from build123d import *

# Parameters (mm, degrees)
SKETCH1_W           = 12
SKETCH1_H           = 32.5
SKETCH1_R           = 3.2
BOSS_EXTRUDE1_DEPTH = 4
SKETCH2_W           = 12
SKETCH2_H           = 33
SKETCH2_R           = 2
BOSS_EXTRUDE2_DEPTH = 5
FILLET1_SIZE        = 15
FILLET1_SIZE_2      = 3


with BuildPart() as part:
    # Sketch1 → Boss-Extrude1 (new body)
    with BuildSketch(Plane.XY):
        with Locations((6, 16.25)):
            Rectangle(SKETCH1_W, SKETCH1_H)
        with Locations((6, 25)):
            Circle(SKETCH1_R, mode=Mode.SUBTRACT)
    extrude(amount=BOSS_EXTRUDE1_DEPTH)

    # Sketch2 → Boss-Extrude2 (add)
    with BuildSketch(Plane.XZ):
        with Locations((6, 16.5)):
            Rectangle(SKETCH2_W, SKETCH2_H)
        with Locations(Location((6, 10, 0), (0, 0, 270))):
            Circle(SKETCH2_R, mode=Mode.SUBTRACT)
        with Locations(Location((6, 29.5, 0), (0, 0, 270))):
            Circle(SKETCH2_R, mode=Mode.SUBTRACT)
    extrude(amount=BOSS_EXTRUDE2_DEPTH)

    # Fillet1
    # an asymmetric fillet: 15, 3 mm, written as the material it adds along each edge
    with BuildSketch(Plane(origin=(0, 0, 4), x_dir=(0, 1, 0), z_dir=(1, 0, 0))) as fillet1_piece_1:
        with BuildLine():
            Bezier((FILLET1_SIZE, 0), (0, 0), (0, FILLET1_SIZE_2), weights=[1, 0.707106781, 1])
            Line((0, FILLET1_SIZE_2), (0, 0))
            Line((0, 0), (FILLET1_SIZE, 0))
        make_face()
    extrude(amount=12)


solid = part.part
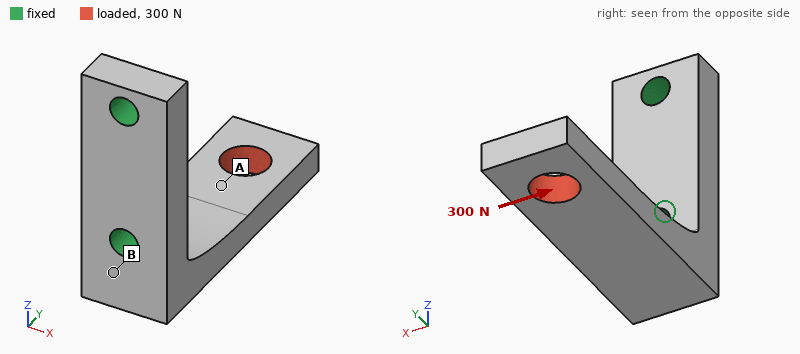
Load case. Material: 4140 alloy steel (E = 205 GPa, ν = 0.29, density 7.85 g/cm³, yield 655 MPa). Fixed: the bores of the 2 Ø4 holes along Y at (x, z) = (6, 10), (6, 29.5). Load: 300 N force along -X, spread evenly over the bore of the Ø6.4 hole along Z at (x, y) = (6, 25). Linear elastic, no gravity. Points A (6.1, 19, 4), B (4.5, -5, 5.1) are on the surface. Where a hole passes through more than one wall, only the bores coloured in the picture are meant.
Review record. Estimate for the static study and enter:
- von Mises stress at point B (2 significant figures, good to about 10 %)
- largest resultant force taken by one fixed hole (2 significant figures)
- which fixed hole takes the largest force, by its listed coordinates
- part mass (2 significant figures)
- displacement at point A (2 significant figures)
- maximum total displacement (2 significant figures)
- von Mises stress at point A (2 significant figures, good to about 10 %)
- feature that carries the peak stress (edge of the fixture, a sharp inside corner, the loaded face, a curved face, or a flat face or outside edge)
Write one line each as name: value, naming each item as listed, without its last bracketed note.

von Mises stress at point B: 74 MPa
largest resultant force taken by one fixed hole: 350 N
which fixed hole takes the largest force, by its listed coordinates: (6, 10)
part mass: 27 g
displacement at point A: 34 µm
maximum total displacement: 62 µm
von Mises stress at point A: 25 MPa
feature that carries the peak stress: edge of the fixture
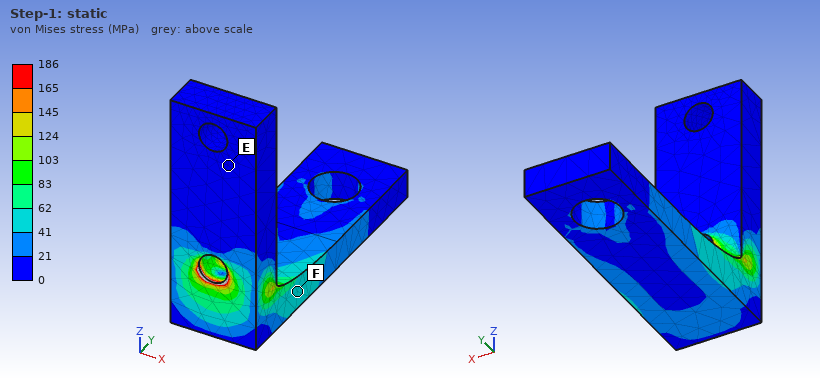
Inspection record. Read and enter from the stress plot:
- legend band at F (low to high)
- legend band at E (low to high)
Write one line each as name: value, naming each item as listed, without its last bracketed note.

legend band at F: 41 to 62 MPa
legend band at E: 0 to 21 MPa
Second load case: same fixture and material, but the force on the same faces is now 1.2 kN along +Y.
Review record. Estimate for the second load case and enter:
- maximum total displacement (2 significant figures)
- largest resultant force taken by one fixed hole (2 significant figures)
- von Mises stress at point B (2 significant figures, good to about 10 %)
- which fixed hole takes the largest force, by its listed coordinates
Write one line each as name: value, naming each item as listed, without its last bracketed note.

maximum total displacement: 52 µm
largest resultant force taken by one fixed hole: 1.3 kN
von Mises stress at point B: 68 MPa
which fixed hole takes the largest force, by its listed coordinates: (6, 10)
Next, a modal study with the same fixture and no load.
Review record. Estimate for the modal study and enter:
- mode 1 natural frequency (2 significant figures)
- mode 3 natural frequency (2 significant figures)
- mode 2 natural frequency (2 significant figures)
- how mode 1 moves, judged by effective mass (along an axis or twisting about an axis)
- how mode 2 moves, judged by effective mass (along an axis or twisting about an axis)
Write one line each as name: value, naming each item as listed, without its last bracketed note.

mode 1 natural frequency: 3200 Hz
mode 3 natural frequency: 13 kHz
mode 2 natural frequency: 5200 Hz
how mode 1 moves, judged by effective mass: along Z
how mode 2 moves, judged by effective mass: along X
